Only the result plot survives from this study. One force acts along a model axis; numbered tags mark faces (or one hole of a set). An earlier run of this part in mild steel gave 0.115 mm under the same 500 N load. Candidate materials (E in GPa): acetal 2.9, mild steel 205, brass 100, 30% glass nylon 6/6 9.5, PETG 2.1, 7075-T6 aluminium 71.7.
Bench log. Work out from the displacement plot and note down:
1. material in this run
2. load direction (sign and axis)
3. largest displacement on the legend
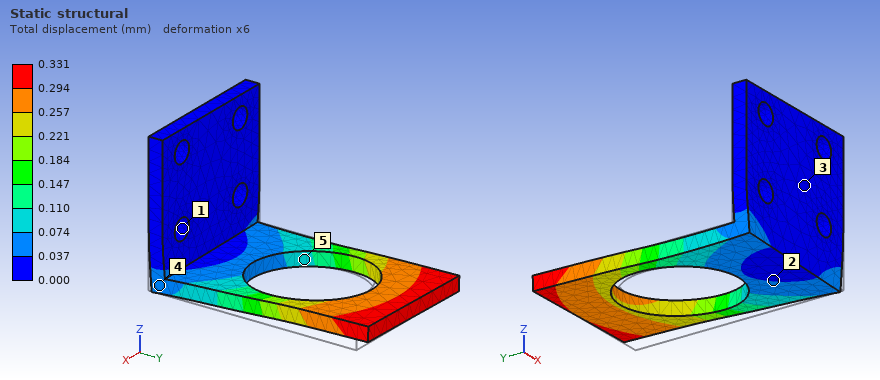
7075-T6 aluminium
-X
0.331 mm
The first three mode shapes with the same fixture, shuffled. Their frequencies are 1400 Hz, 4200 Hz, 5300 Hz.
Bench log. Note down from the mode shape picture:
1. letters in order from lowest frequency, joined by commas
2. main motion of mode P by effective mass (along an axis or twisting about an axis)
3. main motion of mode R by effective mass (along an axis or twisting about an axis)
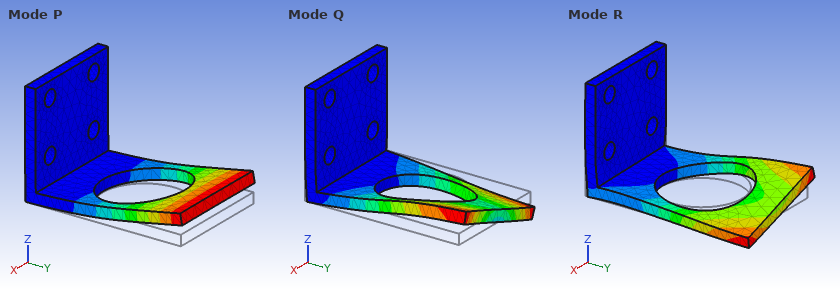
P, Q, R
along Z
along X
